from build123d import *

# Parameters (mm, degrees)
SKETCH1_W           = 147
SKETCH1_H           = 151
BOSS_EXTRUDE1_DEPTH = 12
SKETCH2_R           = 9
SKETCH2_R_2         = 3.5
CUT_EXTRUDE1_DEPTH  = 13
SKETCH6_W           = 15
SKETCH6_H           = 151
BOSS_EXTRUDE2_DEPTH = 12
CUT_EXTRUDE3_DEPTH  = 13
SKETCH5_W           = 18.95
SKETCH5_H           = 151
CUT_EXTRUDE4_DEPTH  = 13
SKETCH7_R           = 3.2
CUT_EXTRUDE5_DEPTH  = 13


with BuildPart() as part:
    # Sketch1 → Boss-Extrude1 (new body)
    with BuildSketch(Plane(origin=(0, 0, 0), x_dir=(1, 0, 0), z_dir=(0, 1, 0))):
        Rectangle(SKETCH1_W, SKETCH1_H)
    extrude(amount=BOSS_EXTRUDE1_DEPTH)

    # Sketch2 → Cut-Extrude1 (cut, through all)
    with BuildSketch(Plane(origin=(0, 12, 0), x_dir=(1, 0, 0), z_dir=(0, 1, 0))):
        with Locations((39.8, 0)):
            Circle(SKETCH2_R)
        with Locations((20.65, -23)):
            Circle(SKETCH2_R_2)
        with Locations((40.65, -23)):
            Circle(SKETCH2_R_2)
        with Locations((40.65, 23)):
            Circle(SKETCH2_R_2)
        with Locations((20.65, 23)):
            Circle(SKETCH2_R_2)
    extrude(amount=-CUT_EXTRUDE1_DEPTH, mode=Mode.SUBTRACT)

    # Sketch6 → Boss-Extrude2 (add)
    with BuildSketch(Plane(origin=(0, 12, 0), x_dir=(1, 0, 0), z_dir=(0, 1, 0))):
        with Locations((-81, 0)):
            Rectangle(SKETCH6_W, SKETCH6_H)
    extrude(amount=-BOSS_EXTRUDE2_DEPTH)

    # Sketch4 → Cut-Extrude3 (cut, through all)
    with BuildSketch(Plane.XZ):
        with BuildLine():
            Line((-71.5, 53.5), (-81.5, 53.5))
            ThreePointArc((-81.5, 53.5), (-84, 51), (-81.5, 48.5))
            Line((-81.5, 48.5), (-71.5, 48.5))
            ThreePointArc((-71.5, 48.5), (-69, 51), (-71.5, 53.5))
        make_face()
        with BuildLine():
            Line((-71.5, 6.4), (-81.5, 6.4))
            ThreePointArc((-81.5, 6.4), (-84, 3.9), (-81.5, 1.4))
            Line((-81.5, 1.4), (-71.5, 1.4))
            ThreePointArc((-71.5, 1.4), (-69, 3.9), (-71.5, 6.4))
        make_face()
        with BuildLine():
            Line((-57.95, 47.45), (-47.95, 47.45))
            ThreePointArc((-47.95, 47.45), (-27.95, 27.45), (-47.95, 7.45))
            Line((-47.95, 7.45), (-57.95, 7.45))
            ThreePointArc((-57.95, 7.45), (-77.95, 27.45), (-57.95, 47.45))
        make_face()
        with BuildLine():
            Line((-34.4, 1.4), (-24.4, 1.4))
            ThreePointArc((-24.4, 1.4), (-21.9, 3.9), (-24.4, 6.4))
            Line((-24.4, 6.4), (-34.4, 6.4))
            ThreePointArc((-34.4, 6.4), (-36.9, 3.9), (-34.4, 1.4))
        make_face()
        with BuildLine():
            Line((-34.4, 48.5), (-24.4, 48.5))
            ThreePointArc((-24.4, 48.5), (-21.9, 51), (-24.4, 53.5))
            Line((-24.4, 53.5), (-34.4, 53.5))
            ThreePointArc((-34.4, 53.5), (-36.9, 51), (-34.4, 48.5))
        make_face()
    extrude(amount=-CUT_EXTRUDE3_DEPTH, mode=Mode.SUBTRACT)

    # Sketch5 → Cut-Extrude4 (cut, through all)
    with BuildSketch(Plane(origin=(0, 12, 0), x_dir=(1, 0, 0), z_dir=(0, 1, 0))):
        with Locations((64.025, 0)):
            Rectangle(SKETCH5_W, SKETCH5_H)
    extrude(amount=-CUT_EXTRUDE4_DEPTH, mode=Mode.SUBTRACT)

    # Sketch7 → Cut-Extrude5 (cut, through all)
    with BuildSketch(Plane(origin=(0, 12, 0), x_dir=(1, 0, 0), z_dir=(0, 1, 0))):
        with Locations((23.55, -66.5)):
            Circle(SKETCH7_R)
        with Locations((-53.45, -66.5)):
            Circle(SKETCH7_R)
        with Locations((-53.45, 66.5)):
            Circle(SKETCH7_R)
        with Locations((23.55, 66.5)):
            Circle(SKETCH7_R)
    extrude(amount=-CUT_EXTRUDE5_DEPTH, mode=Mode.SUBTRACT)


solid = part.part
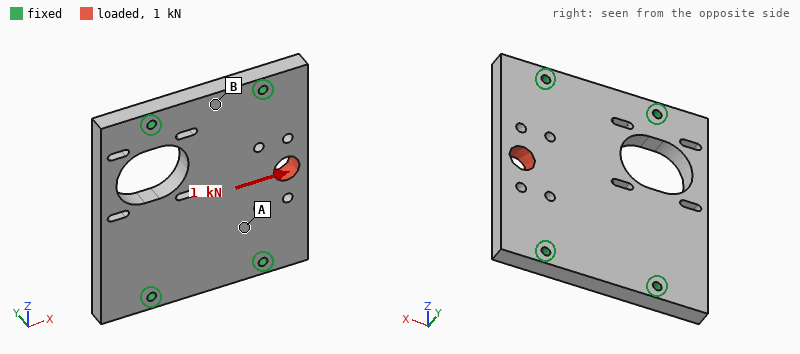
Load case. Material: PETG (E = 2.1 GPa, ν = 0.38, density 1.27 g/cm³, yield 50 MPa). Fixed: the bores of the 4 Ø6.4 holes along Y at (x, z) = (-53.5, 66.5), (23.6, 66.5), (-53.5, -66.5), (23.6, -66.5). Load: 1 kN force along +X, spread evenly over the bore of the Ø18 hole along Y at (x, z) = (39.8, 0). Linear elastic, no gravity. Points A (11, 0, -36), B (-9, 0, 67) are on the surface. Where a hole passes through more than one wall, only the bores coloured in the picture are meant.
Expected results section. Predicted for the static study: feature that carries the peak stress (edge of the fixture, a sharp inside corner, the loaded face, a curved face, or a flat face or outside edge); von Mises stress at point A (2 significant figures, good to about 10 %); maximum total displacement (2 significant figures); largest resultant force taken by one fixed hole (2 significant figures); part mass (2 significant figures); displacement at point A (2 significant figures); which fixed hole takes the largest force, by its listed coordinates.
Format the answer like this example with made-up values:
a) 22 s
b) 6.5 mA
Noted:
a) a flat face or outside edge
b) 1.0 MPa
c) 0.10 mm
d) 340 N
e) 290 g
f) 0.030 mm
g) (-53.5, -66.5)
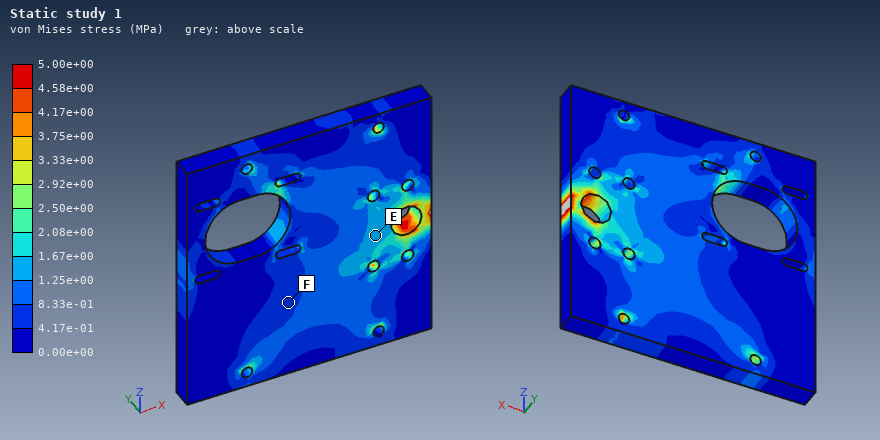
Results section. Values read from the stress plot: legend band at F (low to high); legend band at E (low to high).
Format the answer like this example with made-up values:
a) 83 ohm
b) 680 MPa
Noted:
a) 4.17e-01 to 8.33e-01 MPa
b) 1.25e+00 to 1.67e+00 MPa
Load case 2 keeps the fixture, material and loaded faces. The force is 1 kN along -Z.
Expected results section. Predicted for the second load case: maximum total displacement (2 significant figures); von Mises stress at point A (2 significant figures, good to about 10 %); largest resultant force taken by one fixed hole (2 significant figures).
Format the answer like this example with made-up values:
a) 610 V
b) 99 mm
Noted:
a) 53 µm
b) 0.47 MPa
c) 450 N
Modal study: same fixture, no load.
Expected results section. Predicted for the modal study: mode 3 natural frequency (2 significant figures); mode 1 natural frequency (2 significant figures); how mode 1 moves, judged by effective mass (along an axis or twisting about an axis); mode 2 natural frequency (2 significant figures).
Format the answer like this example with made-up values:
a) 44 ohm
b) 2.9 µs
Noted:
a) 1100 Hz
b) 630 Hz
c) along Y
d) 770 Hz
